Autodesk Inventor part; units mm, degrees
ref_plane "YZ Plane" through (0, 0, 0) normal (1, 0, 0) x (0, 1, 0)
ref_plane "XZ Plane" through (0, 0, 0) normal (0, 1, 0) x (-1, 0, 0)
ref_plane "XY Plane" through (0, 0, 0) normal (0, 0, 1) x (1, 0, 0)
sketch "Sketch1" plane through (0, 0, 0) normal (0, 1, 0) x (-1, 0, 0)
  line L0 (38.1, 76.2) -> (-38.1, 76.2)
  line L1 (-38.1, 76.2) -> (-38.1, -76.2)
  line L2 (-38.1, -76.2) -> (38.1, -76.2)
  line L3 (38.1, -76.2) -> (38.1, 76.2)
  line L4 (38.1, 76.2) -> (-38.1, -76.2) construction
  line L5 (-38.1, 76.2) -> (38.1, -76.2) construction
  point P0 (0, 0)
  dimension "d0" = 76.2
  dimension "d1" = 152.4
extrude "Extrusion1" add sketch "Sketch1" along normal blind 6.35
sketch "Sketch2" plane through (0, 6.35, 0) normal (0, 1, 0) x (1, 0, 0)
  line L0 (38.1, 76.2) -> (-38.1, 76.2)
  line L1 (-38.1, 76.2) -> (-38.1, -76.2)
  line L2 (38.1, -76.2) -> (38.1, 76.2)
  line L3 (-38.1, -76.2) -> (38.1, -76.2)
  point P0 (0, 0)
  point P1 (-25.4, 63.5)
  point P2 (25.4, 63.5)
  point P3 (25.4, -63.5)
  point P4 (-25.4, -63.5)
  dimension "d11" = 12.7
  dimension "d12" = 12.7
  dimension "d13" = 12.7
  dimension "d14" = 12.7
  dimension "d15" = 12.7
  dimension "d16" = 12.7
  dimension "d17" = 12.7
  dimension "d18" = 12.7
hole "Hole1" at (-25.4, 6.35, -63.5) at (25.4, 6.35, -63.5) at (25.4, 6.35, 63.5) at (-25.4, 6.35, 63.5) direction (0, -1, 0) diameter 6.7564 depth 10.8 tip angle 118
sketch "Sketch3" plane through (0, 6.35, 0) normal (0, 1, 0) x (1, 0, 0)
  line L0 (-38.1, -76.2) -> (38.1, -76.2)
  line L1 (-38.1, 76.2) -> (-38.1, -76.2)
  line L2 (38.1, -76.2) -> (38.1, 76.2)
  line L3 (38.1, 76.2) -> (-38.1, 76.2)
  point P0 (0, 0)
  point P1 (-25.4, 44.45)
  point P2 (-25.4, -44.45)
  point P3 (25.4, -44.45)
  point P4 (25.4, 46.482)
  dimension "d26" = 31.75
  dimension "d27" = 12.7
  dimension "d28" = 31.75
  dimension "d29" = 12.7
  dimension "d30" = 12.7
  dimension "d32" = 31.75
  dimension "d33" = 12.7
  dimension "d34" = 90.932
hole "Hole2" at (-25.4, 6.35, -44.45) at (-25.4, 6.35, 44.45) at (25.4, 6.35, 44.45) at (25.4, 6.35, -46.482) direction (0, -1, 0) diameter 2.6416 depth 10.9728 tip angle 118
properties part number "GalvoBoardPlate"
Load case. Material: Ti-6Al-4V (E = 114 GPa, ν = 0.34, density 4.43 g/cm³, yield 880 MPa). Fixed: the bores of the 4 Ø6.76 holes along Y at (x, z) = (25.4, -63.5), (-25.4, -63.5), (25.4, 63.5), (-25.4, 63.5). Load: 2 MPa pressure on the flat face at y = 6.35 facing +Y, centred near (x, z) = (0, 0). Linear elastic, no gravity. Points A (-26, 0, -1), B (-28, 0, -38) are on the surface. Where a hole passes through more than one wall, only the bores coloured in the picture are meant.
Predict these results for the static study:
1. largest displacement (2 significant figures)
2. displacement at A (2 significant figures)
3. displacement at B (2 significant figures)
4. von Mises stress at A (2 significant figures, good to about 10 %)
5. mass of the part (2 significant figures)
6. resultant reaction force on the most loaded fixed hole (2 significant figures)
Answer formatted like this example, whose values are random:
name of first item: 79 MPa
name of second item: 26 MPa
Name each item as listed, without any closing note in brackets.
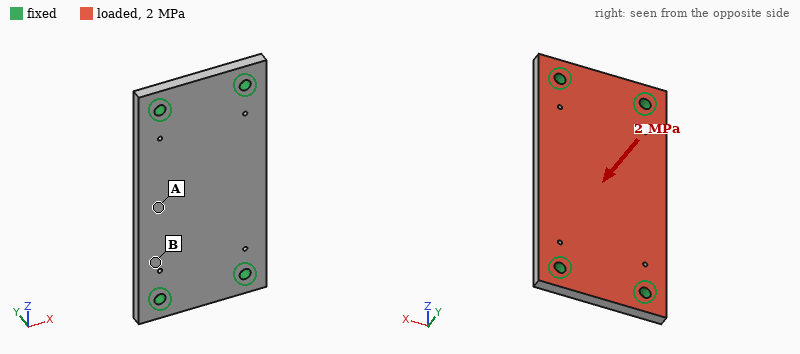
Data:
largest displacement: 0.62 mm
displacement at A: 0.59 mm
displacement at B: 0.26 mm
von Mises stress at A: 200 MPa
mass of the part: 320 g
resultant reaction force on the most loaded fixed hole: 5.7 kN
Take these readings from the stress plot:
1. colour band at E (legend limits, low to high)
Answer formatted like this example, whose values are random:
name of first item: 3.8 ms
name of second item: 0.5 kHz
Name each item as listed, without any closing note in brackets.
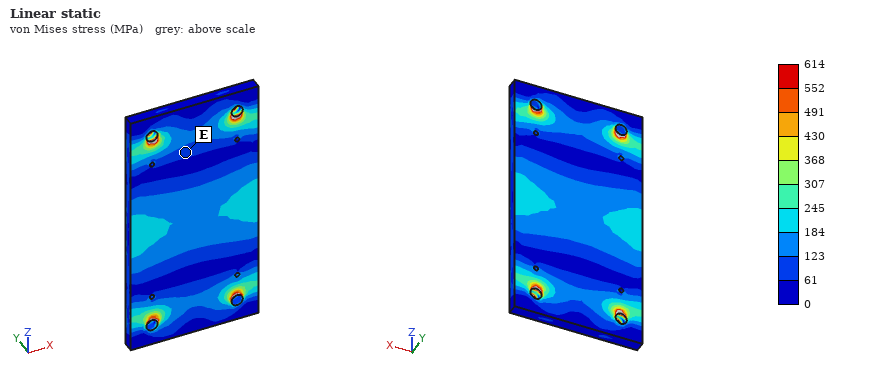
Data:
colour band at E: 61 to 123 MPa
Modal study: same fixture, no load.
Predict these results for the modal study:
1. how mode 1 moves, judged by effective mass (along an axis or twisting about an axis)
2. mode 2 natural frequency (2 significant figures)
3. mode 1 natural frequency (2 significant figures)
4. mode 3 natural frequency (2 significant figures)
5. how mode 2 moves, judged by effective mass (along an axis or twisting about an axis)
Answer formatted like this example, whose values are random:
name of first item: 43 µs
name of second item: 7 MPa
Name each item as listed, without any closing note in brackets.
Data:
how mode 1 moves, judged by effective mass: along Y
mode 2 natural frequency: 3000 Hz
mode 1 natural frequency: 2000 Hz
mode 3 natural frequency: 5400 Hz
how mode 2 moves, judged by effective mass: twisting about Z
